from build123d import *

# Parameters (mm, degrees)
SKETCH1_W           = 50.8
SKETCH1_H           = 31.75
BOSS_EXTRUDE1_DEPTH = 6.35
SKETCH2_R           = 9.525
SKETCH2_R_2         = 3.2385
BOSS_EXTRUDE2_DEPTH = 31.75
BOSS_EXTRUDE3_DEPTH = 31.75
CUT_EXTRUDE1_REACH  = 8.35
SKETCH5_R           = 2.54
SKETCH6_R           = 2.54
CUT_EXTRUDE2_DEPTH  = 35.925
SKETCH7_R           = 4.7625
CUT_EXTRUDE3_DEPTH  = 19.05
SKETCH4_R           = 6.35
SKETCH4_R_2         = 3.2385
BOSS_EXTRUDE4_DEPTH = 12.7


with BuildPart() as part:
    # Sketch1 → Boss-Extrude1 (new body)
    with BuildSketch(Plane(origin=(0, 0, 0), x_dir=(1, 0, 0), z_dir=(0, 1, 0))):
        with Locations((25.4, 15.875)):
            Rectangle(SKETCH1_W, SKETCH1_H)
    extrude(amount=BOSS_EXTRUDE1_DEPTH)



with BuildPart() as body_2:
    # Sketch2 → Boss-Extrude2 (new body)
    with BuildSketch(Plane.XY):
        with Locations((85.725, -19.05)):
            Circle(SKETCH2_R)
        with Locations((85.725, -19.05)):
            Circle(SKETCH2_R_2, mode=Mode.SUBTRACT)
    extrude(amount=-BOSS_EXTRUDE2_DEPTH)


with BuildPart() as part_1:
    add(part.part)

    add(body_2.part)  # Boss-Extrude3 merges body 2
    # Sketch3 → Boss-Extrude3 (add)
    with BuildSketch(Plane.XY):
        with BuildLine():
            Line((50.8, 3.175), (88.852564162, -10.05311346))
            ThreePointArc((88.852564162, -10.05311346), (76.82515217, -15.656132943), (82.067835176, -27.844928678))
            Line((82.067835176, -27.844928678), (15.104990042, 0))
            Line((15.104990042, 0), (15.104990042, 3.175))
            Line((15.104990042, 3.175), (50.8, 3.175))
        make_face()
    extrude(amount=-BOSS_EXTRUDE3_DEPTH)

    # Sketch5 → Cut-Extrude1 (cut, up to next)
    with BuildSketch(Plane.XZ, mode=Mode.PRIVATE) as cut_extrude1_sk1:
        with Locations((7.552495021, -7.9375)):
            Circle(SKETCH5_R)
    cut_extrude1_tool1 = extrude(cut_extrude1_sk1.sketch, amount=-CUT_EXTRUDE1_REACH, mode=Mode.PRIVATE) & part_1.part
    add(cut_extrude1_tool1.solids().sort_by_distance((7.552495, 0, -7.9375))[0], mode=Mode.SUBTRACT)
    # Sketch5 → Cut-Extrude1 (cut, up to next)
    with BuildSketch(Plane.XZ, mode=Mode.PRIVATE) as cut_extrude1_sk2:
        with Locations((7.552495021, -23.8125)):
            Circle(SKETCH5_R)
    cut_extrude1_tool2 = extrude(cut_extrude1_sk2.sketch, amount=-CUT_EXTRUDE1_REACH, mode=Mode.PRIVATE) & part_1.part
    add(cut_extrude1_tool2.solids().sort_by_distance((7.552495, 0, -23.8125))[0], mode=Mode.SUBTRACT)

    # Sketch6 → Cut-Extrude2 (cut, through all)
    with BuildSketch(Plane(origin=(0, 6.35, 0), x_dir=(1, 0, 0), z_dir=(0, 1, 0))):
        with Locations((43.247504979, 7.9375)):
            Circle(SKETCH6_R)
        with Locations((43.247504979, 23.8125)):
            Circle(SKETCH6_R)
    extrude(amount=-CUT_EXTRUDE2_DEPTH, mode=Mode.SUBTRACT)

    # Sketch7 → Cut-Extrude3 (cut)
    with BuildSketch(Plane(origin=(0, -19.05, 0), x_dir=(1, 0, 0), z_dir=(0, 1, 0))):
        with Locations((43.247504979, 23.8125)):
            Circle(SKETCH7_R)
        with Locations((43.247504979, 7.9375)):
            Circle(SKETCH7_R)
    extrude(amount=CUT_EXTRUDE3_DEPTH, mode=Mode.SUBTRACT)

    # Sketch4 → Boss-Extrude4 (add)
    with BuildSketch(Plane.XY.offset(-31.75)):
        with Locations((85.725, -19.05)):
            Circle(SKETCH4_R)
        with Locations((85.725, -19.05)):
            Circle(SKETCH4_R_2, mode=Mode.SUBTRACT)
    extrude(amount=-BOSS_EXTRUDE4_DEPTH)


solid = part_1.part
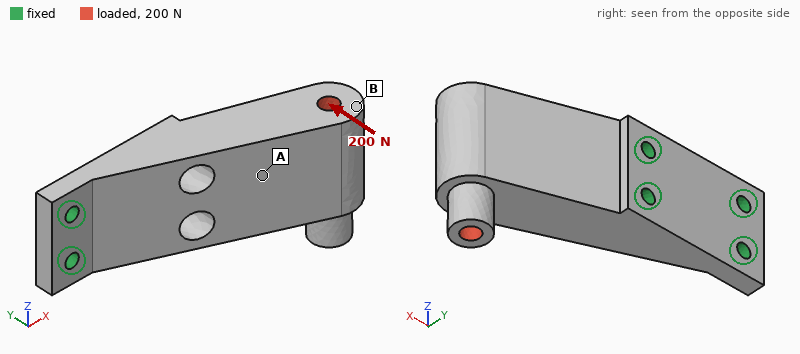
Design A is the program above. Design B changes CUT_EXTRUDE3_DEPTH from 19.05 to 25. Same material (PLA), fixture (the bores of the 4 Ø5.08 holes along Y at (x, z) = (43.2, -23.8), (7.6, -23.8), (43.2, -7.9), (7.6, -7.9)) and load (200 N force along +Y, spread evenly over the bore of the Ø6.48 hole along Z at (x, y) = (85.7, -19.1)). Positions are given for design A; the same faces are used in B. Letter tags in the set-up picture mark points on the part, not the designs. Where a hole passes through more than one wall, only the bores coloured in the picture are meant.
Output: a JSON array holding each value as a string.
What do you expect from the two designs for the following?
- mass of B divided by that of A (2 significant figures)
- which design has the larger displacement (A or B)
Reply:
["0.99", "B"]
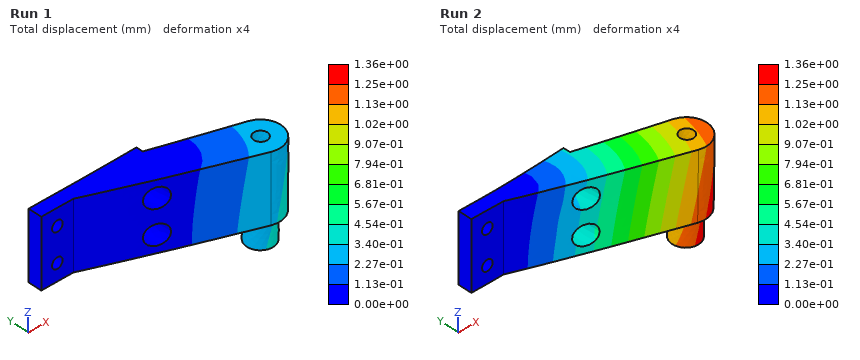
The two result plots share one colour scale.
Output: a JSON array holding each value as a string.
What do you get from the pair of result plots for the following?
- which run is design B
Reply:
["Run 2"]
